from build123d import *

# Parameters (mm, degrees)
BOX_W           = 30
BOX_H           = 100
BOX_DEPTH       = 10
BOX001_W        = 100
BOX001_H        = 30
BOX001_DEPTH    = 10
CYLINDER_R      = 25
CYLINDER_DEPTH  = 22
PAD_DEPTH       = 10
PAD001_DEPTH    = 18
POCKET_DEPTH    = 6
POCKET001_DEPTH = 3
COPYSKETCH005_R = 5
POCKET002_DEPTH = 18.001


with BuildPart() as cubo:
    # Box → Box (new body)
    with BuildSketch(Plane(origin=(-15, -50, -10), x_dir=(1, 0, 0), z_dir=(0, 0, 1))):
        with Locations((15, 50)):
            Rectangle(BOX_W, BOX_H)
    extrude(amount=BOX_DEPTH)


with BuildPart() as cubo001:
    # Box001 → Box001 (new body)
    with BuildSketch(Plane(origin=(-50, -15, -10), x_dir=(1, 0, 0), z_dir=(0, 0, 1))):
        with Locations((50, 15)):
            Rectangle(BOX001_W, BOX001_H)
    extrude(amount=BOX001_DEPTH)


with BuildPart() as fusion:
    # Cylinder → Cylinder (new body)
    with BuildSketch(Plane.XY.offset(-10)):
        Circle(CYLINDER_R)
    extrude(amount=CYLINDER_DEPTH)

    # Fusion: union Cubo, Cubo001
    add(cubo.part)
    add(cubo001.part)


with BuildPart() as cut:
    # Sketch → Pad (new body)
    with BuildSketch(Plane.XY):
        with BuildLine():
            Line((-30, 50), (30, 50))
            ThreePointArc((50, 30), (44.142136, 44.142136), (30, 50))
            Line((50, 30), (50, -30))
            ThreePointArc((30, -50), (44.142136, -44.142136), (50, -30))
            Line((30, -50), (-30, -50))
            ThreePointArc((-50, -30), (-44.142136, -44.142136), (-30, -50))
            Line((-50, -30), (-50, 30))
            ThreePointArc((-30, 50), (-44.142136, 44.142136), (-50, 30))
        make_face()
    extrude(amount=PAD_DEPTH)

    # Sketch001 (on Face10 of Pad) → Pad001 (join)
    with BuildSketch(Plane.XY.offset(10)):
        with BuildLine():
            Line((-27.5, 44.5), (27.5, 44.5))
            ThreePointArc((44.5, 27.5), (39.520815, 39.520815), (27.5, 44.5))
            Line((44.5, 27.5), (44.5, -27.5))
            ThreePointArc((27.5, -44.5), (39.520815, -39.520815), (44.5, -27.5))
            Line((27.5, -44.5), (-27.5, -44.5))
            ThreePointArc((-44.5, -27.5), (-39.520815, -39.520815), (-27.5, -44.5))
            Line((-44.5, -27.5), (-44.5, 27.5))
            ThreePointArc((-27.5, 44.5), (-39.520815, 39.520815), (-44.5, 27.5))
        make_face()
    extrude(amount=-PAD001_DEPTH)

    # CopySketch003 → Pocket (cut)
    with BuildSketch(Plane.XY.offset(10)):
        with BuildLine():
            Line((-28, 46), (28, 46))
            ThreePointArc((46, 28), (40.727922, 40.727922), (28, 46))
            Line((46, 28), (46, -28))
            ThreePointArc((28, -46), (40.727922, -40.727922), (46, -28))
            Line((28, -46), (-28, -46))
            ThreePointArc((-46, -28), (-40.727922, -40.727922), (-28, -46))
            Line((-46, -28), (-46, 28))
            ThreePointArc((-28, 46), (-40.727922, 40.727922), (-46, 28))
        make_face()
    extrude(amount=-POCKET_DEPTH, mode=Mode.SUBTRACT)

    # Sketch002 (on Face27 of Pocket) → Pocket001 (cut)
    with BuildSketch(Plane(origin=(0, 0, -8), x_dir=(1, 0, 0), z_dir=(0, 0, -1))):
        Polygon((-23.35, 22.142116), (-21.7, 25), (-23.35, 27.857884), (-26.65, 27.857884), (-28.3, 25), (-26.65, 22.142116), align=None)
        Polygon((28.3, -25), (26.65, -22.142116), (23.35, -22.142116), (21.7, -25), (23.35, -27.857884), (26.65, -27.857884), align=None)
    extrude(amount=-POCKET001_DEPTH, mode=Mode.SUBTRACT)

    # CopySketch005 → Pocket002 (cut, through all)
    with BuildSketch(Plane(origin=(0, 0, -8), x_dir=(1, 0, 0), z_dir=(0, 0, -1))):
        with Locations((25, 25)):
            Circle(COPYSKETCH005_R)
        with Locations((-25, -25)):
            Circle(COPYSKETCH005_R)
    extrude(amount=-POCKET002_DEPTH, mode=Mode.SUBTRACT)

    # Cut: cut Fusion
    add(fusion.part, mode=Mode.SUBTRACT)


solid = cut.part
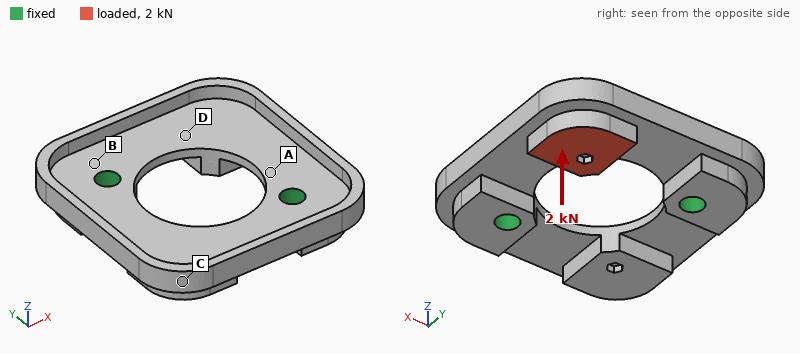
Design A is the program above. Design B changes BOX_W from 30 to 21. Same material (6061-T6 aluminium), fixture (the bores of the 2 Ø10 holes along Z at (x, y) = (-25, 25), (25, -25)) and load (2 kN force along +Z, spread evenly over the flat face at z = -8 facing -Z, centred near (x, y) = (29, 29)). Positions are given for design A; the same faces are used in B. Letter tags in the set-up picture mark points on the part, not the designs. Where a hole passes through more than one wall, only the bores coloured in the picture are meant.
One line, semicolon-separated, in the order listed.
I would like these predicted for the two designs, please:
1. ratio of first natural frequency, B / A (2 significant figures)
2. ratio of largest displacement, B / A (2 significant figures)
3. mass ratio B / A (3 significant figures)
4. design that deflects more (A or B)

1.1; 0.82; 1.05; A
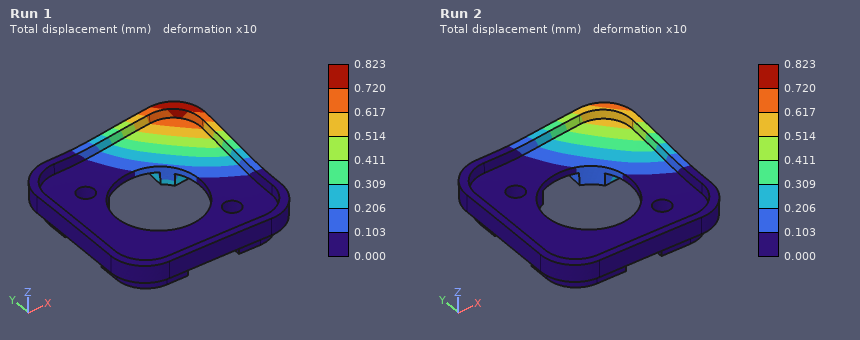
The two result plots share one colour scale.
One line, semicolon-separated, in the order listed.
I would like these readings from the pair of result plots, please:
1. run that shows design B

Run 2
